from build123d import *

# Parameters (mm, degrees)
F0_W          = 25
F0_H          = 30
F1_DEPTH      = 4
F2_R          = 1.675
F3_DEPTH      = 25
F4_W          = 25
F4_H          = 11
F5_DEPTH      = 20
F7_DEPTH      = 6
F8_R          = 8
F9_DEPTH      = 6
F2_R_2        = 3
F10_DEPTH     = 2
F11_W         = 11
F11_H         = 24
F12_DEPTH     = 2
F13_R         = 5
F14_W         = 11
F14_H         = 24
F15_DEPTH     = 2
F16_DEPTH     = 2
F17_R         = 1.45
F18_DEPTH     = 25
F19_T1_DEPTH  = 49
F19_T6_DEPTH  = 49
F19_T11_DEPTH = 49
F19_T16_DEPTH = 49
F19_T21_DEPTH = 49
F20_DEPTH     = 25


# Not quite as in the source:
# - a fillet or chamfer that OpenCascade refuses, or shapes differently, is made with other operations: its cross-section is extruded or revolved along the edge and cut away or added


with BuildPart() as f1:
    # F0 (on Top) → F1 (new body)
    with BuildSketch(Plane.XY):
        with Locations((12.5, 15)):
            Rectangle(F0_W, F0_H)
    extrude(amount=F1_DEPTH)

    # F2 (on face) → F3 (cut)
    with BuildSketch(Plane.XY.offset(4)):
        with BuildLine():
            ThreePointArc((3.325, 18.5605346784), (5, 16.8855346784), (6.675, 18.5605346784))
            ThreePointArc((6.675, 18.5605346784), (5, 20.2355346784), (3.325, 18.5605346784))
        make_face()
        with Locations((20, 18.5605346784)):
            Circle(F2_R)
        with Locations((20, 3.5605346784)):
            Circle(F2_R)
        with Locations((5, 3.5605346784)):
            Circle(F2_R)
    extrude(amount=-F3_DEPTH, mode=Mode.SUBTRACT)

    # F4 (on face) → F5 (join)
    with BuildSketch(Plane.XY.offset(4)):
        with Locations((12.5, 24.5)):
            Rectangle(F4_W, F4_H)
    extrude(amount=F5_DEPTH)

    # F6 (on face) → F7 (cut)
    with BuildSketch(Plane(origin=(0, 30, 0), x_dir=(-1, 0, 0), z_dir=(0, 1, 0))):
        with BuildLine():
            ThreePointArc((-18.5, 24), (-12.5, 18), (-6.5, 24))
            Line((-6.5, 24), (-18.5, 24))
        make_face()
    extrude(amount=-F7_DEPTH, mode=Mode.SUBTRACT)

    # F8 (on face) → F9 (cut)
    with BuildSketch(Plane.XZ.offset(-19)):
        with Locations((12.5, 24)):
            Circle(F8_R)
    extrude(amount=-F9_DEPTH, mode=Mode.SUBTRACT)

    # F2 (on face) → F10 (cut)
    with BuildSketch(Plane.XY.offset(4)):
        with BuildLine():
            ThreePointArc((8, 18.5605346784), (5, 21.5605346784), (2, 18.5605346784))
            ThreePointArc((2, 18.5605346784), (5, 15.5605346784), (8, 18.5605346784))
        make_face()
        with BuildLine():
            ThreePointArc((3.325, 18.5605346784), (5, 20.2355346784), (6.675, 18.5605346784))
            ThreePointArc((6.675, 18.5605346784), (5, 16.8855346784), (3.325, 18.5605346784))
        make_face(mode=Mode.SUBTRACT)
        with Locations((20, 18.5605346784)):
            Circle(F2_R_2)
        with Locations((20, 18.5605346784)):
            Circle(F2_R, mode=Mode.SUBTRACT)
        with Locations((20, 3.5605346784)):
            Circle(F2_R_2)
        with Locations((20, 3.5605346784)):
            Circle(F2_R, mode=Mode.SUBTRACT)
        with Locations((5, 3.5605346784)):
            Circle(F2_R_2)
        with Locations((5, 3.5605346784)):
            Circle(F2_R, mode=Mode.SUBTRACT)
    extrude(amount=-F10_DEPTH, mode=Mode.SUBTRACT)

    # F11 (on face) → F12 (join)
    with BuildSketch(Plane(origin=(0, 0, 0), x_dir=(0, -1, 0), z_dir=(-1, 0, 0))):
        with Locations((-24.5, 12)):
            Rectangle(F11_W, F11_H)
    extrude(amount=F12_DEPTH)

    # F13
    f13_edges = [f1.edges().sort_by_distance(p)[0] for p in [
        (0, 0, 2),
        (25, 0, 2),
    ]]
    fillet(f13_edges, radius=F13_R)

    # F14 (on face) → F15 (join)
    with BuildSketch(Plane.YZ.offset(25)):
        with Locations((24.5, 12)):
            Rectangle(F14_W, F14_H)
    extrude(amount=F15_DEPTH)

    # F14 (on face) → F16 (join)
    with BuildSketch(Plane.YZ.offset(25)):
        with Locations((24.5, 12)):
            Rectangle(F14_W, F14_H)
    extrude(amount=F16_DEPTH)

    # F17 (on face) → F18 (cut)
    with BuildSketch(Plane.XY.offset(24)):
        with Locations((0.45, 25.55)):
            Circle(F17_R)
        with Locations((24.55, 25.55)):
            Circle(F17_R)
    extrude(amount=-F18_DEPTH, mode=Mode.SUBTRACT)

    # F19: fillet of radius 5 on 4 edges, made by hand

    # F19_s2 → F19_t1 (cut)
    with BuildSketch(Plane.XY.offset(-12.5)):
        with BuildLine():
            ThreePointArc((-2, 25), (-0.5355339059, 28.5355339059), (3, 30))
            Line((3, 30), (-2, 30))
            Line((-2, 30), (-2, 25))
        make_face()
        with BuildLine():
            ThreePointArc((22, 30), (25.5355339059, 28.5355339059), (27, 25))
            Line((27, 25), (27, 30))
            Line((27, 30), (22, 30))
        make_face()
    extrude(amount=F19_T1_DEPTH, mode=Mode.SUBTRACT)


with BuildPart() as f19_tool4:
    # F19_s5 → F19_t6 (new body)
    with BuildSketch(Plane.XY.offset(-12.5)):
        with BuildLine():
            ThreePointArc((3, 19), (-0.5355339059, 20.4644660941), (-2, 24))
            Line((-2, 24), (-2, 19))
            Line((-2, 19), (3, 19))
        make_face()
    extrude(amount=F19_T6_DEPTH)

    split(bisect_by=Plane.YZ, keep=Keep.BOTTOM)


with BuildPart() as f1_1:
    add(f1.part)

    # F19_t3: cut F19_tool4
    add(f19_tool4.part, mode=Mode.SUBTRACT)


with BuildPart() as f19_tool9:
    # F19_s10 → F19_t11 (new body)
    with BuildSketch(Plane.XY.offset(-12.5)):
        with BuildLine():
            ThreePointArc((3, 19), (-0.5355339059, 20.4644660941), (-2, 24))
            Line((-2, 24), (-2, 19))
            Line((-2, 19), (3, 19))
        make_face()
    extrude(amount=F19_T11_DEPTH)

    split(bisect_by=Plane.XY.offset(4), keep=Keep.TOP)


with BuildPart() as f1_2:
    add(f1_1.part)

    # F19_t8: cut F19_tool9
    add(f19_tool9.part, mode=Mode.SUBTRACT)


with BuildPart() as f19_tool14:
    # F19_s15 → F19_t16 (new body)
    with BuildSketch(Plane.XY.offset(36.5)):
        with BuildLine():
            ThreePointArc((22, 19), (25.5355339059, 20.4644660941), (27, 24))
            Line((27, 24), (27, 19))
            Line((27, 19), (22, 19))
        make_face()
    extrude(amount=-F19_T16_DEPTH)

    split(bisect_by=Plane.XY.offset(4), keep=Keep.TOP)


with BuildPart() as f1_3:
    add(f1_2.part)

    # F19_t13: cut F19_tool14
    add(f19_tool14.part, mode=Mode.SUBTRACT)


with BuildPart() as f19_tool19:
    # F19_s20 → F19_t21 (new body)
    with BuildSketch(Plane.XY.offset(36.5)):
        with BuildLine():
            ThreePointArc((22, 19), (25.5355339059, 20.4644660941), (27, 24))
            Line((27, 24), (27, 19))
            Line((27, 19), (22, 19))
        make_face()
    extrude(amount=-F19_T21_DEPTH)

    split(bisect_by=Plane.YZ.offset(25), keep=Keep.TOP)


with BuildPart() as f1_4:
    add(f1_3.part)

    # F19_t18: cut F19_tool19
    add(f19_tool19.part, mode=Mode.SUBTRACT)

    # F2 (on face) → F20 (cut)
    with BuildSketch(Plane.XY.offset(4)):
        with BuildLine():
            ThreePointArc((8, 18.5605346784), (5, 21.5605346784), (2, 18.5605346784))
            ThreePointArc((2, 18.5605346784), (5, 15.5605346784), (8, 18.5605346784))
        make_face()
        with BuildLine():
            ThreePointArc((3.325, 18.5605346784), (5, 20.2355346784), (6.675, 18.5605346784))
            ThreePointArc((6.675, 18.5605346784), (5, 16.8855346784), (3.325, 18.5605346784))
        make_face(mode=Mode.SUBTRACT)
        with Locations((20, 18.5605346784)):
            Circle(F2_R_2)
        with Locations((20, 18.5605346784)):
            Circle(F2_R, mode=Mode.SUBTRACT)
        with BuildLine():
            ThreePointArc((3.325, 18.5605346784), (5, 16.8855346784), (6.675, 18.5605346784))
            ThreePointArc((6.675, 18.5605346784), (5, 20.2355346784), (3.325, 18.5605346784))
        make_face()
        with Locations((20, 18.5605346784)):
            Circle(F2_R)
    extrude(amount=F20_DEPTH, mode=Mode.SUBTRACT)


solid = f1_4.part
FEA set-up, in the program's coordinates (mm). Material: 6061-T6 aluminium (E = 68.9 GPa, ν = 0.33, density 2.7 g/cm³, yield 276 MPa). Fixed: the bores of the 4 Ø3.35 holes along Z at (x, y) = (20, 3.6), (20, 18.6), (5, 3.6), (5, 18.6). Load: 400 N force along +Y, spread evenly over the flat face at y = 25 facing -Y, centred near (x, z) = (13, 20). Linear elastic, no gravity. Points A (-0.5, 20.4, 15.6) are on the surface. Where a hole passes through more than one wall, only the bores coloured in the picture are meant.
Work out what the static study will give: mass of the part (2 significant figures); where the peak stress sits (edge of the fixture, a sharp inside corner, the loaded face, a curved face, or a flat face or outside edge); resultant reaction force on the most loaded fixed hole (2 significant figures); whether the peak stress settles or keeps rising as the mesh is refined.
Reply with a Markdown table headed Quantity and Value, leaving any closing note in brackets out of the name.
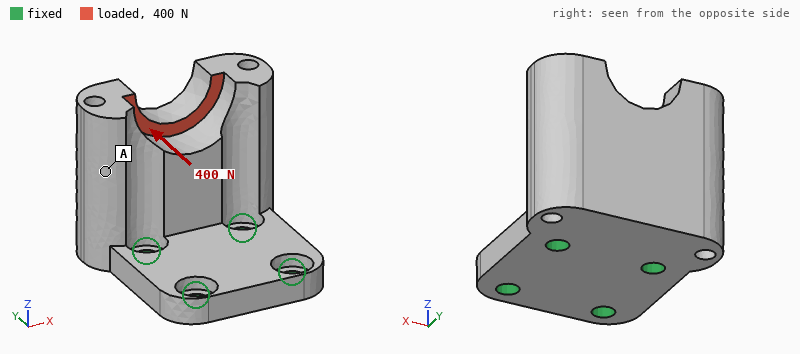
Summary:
| Quantity | Value |
|---|---|
| mass of the part | 19 g |
| where the peak stress sits | edge of the fixture |
| resultant reaction force on the most loaded fixed hole | 360 N |
| whether the peak stress settles or keeps rising as the mesh is refined | keeps rising |
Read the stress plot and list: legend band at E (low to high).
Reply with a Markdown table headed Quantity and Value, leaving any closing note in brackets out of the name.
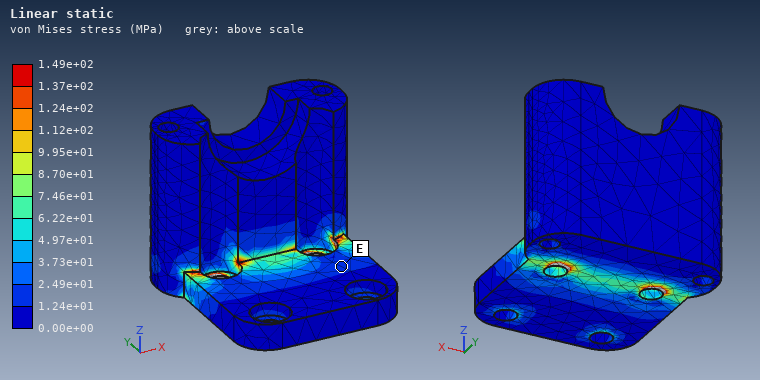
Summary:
| Quantity | Value |
|---|---|
| legend band at E | 1.24e+01 to 2.49e+01 MPa |
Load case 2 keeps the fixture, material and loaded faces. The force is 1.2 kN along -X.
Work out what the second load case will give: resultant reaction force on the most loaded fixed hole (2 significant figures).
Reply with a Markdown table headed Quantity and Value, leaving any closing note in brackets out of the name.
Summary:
| Quantity | Value |
|---|---|
| resultant reaction force on the most loaded fixed hole | 1.5 kN |
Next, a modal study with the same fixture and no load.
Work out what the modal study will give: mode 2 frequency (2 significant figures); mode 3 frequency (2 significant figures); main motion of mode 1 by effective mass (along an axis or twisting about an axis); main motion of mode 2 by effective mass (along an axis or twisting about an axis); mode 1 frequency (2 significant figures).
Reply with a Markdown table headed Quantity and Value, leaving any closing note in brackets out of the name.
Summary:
| Quantity | Value |
|---|---|
| mode 2 frequency | 10 kHz |
| mode 3 frequency | 17 kHz |
| main motion of mode 1 by effective mass | along Y |
| main motion of mode 2 by effective mass | along X |
| mode 1 frequency | 4300 Hz |
